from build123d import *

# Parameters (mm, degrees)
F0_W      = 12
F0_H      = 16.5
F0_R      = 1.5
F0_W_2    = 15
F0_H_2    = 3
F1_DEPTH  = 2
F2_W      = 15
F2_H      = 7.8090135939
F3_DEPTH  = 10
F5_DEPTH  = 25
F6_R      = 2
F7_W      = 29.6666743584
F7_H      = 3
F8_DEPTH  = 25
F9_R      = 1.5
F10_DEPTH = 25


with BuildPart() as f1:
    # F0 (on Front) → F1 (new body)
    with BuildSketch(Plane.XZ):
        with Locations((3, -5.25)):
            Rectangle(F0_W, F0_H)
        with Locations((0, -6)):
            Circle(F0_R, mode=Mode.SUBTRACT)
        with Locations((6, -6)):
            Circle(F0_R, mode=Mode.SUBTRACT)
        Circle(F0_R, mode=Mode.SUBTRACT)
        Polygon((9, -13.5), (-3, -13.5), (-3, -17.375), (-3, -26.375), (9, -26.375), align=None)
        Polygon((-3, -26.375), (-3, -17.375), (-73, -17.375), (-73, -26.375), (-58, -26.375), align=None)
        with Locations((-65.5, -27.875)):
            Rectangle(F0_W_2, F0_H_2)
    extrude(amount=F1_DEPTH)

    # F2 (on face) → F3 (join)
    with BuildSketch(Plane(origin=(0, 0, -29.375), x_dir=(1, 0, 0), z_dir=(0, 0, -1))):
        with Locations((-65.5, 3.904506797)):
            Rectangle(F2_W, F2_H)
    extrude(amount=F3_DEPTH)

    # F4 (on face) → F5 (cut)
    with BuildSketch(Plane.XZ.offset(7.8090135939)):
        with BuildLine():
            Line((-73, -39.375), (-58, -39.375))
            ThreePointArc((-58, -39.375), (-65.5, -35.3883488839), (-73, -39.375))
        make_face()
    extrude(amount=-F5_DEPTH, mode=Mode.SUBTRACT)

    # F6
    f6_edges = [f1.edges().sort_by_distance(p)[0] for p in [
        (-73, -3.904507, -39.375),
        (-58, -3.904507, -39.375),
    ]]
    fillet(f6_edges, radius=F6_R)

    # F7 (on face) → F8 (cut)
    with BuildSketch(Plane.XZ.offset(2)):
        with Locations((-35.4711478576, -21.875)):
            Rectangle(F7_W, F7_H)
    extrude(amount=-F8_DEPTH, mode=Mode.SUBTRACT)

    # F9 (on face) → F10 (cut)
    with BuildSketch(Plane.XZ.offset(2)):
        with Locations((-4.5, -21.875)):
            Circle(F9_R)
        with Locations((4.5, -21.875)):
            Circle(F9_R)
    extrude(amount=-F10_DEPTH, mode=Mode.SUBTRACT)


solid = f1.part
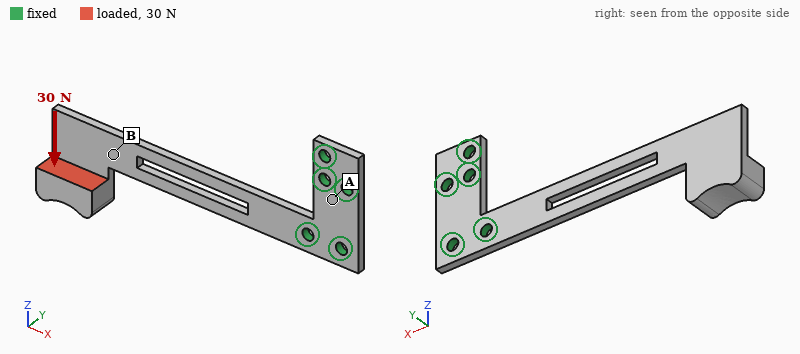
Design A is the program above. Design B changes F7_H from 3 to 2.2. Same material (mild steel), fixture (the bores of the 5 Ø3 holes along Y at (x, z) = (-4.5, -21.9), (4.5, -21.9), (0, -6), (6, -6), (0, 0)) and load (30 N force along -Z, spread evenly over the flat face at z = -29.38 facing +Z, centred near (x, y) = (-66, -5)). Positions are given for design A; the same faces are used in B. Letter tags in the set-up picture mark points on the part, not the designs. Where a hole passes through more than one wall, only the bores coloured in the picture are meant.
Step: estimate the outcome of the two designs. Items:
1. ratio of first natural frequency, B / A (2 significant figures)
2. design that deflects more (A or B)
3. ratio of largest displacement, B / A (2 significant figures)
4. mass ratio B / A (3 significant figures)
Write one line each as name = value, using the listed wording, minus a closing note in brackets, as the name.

ratio of first natural frequency, B / A = 1.0
design that deflects more = A
ratio of largest displacement, B / A = 0.90
mass ratio B / A = 1.02
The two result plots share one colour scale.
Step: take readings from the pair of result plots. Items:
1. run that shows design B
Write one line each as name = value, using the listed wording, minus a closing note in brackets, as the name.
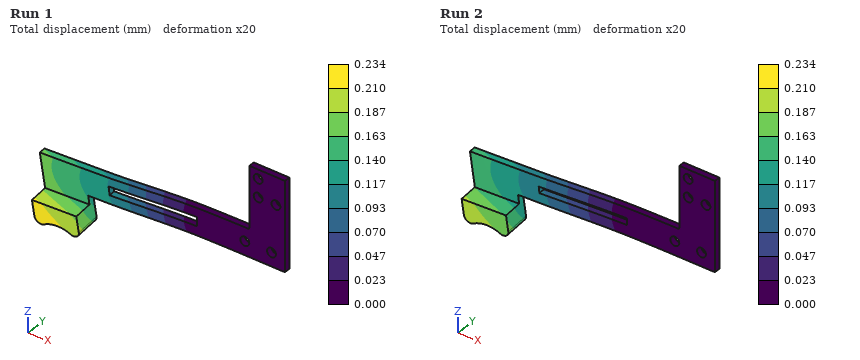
run that shows design B = Run 2
